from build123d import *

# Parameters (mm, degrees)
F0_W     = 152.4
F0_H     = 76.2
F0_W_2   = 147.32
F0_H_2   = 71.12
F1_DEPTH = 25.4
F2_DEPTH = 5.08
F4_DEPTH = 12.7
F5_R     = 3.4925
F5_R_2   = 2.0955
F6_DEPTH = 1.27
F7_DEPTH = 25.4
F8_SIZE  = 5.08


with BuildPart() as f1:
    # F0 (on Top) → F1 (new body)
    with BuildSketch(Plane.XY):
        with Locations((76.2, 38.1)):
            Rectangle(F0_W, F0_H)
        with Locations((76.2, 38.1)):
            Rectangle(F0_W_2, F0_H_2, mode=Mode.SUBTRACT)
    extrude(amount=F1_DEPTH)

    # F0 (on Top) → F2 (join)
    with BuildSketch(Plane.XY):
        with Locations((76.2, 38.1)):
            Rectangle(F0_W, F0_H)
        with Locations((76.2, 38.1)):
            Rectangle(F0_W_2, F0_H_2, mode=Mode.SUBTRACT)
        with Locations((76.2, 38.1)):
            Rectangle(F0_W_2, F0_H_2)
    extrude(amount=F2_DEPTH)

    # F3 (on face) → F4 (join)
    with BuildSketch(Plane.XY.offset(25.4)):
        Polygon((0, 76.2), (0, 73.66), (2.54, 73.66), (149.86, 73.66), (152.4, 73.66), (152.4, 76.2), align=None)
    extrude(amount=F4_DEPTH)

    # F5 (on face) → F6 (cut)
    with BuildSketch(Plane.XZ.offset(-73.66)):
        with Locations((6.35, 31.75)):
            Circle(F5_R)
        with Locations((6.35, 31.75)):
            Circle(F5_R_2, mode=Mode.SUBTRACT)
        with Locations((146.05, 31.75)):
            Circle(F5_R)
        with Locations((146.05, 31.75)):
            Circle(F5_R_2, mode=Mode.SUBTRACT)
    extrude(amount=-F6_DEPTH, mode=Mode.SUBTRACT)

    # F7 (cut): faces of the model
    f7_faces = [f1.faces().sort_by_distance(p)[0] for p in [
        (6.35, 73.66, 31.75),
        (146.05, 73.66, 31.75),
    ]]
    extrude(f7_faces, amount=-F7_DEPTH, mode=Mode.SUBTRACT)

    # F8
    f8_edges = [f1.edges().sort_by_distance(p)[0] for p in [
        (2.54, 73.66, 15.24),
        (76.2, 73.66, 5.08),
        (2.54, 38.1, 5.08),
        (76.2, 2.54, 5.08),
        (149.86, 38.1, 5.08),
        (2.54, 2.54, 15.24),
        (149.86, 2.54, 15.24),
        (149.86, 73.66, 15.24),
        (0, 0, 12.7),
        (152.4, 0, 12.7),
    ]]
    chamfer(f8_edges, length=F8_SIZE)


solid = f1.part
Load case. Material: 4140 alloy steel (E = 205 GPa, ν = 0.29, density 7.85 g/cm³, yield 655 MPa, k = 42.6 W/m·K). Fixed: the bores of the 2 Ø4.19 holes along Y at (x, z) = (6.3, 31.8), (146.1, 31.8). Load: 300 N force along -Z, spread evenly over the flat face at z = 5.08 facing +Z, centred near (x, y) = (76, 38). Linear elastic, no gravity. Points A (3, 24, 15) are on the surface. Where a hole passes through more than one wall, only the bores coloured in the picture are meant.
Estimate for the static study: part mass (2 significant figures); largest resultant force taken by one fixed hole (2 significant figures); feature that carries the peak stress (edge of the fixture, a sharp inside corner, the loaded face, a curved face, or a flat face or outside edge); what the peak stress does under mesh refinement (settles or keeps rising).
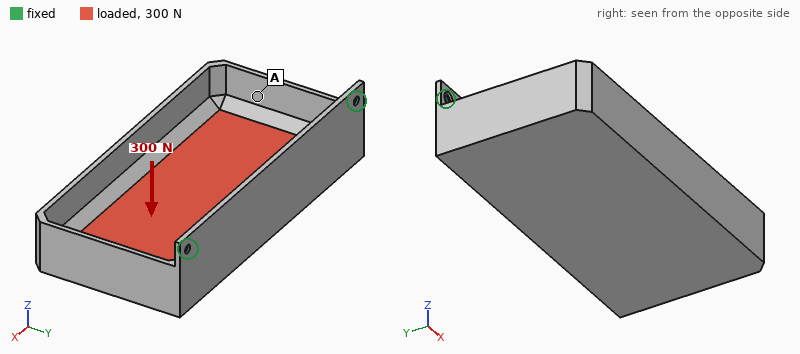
730 g
160 N
edge of the fixture
keeps rising
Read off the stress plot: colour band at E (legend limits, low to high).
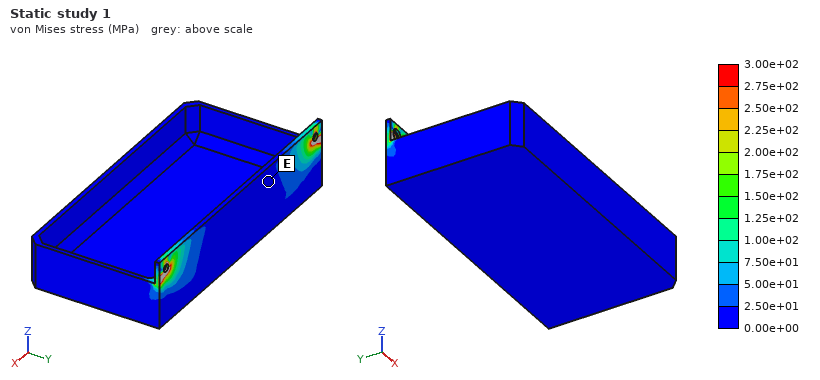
0.00e+00 to 2.50e+01 MPa
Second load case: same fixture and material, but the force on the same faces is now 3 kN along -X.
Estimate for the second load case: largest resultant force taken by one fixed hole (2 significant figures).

1.8 kN
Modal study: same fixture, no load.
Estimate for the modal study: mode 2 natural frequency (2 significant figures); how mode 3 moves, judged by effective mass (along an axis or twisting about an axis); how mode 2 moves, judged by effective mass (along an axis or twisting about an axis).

530 Hz
along Y
along X
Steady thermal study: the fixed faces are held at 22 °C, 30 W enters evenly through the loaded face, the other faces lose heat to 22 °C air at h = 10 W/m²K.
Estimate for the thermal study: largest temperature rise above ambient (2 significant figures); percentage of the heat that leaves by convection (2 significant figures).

64 K
64 %
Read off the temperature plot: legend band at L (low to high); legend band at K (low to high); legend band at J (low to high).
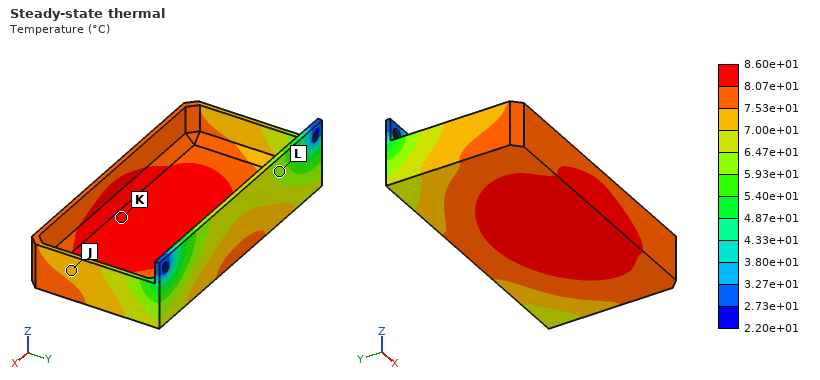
5.93e+01 to 6.47e+01 °C
8.07e+01 to 8.60e+01 °C
7.00e+01 to 7.53e+01 °C
